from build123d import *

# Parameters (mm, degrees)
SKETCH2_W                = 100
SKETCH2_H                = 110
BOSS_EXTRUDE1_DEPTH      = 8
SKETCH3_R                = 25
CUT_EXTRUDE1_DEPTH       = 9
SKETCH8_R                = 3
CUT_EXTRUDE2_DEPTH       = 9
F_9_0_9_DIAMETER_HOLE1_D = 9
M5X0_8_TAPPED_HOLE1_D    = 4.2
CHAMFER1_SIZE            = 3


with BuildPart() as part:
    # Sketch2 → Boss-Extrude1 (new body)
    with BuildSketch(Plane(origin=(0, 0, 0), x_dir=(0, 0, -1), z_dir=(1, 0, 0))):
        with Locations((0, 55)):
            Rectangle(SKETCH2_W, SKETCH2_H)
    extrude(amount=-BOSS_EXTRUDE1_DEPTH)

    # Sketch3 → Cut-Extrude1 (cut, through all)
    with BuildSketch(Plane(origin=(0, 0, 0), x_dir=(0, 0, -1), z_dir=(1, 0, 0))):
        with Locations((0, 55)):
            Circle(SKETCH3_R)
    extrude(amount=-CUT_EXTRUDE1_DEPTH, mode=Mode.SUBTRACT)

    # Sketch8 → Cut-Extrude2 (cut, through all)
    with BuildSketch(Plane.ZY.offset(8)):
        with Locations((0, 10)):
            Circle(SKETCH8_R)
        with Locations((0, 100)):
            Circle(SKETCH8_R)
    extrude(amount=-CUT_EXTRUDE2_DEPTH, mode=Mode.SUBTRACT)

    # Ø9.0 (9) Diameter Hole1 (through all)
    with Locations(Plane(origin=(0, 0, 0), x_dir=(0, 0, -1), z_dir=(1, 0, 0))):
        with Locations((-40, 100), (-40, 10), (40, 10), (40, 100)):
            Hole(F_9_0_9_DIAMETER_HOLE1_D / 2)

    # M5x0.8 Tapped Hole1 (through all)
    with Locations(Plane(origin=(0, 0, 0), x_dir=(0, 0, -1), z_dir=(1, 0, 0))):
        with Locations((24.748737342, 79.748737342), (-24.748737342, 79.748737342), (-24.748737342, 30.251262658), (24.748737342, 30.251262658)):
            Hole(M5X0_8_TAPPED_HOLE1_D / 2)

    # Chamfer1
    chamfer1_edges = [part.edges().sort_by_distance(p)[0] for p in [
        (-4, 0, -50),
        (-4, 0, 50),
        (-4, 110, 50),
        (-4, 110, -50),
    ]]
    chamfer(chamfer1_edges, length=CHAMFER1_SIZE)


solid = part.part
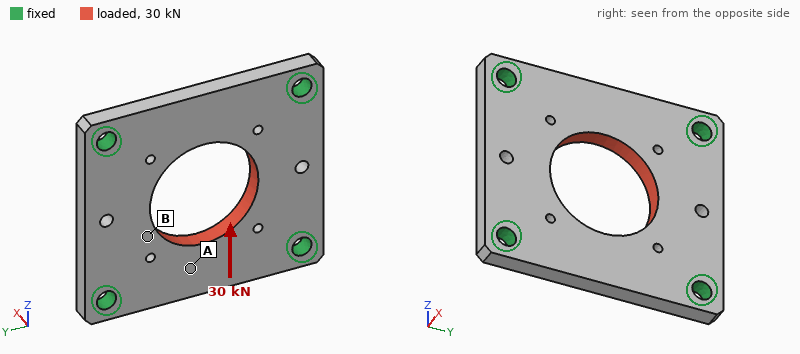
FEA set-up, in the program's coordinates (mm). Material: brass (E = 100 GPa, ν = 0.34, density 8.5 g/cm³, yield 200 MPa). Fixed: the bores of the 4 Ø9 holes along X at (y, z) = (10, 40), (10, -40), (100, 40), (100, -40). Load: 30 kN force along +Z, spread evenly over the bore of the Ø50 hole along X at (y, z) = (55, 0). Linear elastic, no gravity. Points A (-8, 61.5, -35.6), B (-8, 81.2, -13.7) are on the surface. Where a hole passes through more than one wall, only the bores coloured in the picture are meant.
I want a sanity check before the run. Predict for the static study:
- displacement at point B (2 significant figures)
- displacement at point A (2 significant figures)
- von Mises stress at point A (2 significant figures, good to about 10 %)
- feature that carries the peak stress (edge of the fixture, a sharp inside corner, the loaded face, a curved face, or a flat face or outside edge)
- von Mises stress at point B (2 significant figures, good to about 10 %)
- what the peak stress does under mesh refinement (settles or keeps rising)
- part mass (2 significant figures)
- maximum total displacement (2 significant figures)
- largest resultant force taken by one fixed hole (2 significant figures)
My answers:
15 µm
27 µm
20 MPa
edge of the fixture
44 MPa
keeps rising
590 g
30 µm
8.2 kN
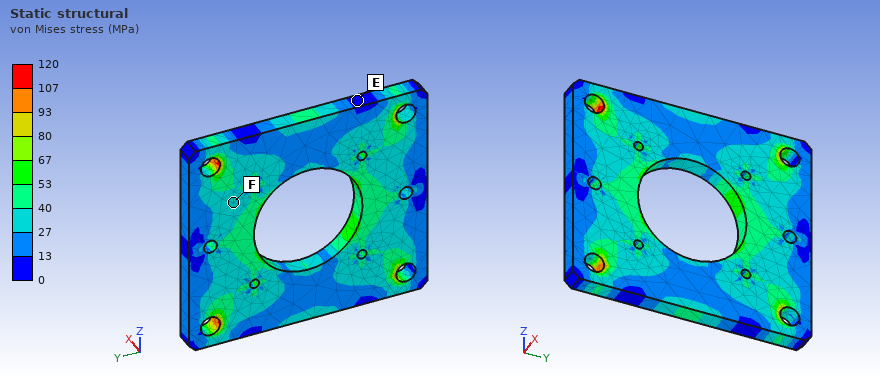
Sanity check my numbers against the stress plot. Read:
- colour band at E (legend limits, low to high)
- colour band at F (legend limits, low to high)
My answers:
0 to 13 MPa
27 to 40 MPa
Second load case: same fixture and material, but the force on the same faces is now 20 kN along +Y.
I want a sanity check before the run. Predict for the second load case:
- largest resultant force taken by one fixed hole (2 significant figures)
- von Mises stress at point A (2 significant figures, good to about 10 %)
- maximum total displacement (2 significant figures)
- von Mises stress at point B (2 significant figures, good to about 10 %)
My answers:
5.4 kN
19 MPa
15 µm
16 MPa
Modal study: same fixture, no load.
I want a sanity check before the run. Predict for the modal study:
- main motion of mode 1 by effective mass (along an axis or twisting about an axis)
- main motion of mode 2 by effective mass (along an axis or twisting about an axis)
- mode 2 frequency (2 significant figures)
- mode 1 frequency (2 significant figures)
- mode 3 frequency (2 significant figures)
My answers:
along X
twisting about Y
3900 Hz
3300 Hz
4500 Hz
